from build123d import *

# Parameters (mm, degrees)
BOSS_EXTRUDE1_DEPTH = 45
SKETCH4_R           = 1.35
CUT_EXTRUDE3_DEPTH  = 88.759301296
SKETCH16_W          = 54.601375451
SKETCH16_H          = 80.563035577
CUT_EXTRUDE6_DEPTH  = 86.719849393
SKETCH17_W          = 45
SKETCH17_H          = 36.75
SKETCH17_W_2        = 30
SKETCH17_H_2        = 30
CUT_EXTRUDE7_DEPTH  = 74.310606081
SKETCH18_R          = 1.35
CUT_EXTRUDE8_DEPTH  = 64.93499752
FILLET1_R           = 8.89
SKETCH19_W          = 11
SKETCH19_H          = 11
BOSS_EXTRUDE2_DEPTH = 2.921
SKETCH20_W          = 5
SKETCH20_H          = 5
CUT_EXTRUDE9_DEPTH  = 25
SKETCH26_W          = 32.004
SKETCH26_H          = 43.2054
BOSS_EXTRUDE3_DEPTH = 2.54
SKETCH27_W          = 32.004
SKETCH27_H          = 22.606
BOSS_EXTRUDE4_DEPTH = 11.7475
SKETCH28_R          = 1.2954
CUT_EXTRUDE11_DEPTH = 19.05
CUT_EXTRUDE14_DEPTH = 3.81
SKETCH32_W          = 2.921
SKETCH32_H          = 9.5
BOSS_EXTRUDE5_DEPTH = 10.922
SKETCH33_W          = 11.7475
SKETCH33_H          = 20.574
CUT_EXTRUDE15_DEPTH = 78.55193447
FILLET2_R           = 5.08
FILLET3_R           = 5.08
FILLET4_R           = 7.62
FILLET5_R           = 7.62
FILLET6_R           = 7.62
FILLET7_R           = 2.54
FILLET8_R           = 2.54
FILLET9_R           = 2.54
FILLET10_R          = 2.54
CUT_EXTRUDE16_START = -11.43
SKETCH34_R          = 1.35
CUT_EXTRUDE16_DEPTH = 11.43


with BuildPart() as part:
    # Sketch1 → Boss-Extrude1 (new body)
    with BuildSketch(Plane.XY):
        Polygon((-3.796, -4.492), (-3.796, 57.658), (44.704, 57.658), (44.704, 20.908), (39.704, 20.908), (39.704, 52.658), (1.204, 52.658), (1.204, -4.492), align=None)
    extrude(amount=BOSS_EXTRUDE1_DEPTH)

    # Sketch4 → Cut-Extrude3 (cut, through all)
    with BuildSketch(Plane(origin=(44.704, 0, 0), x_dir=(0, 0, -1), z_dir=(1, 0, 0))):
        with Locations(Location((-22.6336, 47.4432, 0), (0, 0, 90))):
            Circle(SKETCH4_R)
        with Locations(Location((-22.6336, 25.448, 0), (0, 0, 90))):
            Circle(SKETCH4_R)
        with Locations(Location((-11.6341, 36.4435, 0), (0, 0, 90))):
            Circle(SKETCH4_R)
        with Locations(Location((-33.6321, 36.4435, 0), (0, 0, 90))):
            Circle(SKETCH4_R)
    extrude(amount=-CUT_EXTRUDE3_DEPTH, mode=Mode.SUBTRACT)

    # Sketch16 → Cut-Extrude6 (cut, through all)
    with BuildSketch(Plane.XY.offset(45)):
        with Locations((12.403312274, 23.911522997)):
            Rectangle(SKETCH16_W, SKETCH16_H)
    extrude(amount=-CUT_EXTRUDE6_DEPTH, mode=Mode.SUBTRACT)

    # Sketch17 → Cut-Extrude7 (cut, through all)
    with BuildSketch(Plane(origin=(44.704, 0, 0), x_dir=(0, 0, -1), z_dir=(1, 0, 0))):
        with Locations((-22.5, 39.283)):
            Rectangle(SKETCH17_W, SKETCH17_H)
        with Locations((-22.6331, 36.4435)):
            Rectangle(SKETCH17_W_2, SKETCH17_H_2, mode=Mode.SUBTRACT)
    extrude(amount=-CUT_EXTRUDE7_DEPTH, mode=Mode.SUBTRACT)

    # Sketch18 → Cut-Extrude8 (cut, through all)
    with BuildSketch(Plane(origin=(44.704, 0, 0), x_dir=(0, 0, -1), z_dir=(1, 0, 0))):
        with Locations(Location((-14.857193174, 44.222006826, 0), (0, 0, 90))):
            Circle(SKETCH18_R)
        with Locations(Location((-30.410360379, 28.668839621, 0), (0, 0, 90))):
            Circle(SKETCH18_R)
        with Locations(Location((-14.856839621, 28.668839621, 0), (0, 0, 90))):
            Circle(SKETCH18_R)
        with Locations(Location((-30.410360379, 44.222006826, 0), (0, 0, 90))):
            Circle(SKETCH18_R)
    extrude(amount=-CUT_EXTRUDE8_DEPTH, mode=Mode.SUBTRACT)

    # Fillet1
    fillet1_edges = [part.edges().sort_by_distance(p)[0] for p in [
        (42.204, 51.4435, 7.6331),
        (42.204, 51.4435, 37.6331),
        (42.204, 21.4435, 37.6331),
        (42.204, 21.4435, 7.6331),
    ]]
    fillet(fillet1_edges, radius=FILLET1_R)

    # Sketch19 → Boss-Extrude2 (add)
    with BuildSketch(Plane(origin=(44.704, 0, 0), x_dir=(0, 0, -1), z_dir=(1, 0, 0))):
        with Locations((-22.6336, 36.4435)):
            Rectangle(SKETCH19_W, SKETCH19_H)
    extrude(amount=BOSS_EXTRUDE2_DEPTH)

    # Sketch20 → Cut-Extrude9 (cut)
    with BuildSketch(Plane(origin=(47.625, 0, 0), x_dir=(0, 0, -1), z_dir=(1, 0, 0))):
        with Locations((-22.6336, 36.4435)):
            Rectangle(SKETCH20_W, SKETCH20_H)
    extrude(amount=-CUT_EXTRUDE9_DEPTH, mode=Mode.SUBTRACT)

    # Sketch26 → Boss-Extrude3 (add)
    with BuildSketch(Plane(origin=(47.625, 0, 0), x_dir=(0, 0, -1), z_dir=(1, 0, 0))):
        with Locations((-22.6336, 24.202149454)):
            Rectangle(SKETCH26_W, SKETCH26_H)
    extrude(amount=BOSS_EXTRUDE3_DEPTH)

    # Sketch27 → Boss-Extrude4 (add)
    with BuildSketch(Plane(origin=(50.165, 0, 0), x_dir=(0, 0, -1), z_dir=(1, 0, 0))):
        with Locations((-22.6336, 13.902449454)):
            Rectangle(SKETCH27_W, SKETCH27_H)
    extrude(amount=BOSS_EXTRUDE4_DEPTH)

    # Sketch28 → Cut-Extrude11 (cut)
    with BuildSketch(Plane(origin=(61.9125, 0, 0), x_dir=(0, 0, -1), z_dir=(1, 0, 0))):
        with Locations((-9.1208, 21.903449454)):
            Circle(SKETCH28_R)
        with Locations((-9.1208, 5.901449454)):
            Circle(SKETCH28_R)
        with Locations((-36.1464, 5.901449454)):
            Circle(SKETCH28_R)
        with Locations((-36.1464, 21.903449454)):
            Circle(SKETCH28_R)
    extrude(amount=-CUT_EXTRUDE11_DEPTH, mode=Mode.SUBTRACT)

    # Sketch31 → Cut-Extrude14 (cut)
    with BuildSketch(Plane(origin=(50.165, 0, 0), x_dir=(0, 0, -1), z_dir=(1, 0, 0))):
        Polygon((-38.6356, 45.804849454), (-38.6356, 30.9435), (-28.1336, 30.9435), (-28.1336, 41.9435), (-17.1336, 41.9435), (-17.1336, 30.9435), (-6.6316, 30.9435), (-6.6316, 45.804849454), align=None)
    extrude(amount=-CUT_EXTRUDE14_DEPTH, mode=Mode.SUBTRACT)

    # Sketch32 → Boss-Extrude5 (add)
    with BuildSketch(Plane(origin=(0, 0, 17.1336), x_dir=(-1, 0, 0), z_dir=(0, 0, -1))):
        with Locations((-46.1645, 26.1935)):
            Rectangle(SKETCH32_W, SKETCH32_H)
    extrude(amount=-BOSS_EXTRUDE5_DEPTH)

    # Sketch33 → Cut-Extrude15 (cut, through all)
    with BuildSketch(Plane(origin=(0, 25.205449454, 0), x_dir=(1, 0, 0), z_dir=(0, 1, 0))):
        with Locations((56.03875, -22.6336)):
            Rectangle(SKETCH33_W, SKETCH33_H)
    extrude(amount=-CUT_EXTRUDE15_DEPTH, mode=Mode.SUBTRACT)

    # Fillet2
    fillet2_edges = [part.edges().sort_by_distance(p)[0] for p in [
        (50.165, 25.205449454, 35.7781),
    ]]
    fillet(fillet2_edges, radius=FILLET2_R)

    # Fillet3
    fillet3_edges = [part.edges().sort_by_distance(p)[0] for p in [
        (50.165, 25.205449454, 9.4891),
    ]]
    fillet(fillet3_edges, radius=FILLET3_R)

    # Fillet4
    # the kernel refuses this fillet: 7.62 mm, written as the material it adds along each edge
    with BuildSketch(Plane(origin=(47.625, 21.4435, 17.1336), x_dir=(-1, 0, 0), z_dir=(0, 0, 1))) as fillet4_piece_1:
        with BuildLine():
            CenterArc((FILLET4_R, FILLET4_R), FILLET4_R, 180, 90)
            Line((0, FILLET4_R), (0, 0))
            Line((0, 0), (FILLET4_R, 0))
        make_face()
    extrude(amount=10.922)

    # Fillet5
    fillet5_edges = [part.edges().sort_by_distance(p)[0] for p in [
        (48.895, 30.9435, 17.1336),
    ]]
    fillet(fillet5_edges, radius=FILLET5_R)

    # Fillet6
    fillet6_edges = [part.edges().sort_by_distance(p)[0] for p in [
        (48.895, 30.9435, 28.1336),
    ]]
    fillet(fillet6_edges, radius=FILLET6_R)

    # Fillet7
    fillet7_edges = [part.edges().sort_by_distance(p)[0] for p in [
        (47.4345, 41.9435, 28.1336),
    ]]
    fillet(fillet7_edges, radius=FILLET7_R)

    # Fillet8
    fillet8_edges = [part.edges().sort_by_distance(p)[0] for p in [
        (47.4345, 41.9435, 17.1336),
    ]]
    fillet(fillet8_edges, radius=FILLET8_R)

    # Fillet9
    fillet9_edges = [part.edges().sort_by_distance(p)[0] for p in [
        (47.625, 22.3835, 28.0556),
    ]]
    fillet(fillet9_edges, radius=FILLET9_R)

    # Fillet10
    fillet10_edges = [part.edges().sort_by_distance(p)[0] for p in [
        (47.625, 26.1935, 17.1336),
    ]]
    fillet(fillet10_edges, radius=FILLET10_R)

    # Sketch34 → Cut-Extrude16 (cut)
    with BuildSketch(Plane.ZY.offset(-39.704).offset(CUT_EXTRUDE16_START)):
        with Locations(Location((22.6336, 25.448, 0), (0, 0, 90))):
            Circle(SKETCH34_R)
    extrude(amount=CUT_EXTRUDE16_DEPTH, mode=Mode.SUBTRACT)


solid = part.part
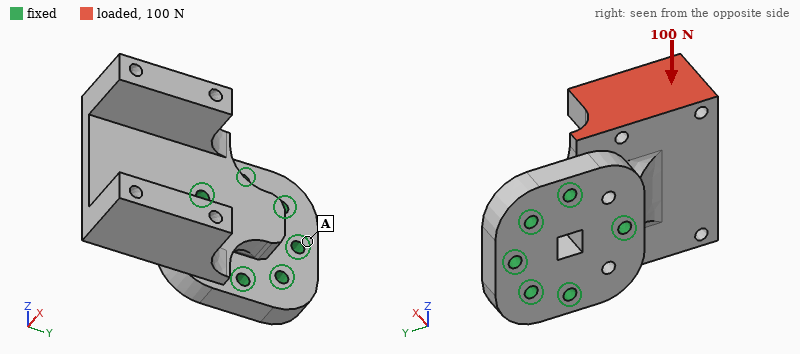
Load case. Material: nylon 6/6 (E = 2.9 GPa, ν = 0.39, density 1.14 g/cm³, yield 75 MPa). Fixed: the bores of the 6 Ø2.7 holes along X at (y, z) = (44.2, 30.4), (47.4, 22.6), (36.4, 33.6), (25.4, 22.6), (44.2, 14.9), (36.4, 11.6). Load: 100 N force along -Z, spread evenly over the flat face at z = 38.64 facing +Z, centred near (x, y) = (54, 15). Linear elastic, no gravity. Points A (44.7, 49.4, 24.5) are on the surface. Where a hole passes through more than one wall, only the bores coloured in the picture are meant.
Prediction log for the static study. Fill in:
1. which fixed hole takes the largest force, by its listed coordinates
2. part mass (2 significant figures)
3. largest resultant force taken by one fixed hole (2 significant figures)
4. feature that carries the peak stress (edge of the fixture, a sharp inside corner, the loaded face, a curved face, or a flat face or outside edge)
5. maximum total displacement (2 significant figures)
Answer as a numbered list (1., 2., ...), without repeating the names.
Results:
1. (25.4, 22.6)
2. 11 g
3. 130 N
4. a curved face
5. 0.72 mm
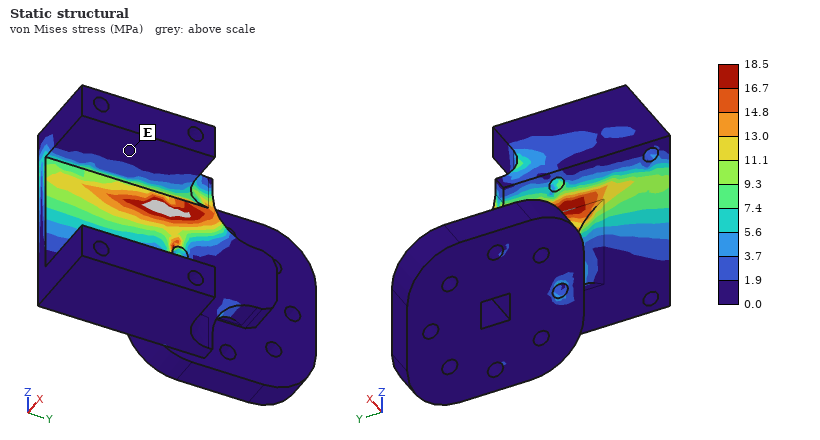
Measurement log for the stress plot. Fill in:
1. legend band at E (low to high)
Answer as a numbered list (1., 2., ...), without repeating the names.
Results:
1. 0.0 to 1.9 MPa
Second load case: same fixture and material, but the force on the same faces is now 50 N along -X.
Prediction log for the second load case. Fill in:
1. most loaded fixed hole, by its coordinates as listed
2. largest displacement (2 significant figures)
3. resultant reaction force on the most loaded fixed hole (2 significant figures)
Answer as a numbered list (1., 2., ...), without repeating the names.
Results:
1. (25.4, 22.6)
2. 0.64 mm
3. 61 N
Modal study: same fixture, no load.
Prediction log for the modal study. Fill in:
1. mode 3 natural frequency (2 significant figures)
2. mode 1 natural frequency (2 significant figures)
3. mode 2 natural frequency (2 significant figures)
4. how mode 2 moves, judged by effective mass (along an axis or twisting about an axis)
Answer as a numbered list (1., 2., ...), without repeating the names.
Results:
1. 2100 Hz
2. 1200 Hz
3. 1400 Hz
4. along X
